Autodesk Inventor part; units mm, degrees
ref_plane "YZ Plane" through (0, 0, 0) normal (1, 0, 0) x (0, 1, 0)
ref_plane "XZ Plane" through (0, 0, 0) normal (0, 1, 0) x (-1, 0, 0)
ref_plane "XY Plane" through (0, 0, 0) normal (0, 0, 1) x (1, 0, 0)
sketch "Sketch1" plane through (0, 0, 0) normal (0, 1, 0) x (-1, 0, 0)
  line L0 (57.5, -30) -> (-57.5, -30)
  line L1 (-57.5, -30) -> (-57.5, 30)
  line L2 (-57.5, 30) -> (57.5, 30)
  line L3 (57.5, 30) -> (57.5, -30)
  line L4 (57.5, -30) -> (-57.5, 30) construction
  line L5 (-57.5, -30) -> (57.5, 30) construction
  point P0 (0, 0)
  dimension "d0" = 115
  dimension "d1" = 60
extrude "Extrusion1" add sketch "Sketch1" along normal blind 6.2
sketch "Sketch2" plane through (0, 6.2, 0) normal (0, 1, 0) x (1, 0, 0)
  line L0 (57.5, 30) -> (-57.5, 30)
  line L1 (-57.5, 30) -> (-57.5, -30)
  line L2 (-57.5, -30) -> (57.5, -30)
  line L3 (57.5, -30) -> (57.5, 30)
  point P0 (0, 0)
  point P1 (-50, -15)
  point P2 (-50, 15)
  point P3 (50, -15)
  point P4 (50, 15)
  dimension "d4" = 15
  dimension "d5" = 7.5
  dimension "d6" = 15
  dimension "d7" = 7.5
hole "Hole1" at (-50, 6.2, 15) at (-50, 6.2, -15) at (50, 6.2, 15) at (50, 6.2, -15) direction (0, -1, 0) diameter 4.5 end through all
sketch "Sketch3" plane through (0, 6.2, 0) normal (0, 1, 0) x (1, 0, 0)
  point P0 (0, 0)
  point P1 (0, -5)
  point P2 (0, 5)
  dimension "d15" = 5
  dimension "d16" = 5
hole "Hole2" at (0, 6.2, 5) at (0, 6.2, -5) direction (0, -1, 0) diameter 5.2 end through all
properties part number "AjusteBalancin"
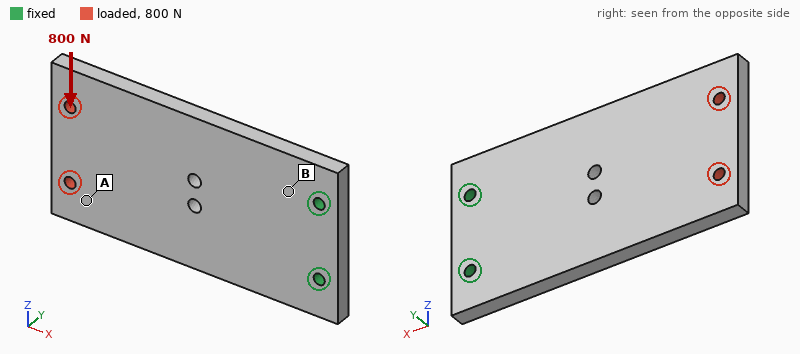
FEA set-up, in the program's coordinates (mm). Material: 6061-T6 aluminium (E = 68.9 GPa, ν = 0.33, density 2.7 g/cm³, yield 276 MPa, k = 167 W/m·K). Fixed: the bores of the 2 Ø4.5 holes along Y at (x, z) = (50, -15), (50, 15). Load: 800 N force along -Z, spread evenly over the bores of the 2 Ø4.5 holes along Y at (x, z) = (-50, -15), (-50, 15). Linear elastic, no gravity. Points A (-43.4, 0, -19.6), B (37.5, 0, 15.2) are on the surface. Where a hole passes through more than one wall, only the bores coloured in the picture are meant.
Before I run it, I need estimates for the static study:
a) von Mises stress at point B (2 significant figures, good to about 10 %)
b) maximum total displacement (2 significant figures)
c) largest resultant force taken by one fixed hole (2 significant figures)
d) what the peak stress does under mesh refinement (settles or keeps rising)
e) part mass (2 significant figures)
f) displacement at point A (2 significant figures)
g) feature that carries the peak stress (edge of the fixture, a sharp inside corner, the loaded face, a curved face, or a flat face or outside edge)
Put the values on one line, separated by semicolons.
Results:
18 MPa; 75 µm; 2.5 kN; keeps rising; 110 g; 63 µm; edge of the fixture
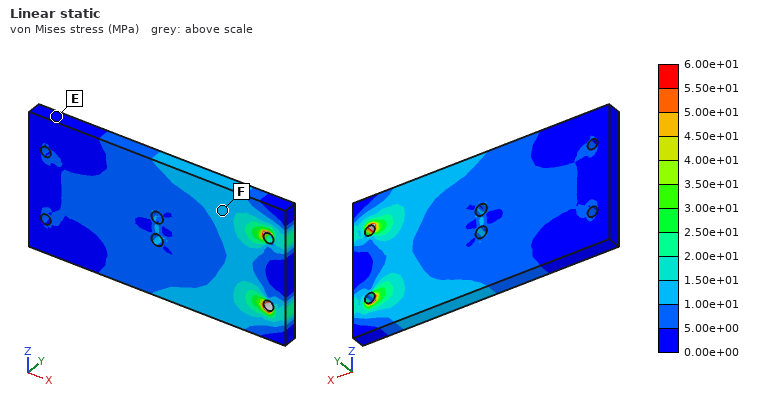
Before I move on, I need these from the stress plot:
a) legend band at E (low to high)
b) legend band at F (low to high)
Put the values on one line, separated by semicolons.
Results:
0.00e+00 to 5.00e+00 MPa; 1.00e+01 to 1.50e+01 MPa
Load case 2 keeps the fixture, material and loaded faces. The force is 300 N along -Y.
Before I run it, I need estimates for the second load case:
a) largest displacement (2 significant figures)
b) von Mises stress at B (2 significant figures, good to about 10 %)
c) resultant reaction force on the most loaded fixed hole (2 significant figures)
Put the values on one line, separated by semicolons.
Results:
1.4 mm; 65 MPa; 150 N
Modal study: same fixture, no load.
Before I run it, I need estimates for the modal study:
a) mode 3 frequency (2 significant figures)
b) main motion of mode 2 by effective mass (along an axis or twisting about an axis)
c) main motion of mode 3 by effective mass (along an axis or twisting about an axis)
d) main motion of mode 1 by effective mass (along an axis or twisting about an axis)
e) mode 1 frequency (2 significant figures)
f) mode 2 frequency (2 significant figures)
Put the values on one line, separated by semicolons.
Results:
2600 Hz; twisting about X; along Y; along Y; 430 Hz; 1600 Hz
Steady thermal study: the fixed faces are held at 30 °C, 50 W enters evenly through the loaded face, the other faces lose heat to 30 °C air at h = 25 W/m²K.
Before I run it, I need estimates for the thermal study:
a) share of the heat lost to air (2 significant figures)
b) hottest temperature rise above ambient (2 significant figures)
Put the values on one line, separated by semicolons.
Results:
27 %; 73 K
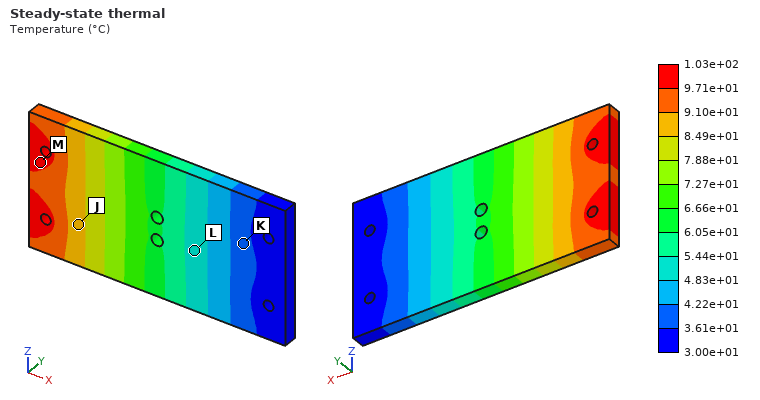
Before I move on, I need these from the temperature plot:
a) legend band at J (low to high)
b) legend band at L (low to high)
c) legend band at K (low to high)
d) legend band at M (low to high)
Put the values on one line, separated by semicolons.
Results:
8.49e+01 to 9.10e+01 °C; 4.83e+01 to 5.44e+01 °C; 3.61e+01 to 4.22e+01 °C; 9.71e+01 to 1.03e+02 °C
